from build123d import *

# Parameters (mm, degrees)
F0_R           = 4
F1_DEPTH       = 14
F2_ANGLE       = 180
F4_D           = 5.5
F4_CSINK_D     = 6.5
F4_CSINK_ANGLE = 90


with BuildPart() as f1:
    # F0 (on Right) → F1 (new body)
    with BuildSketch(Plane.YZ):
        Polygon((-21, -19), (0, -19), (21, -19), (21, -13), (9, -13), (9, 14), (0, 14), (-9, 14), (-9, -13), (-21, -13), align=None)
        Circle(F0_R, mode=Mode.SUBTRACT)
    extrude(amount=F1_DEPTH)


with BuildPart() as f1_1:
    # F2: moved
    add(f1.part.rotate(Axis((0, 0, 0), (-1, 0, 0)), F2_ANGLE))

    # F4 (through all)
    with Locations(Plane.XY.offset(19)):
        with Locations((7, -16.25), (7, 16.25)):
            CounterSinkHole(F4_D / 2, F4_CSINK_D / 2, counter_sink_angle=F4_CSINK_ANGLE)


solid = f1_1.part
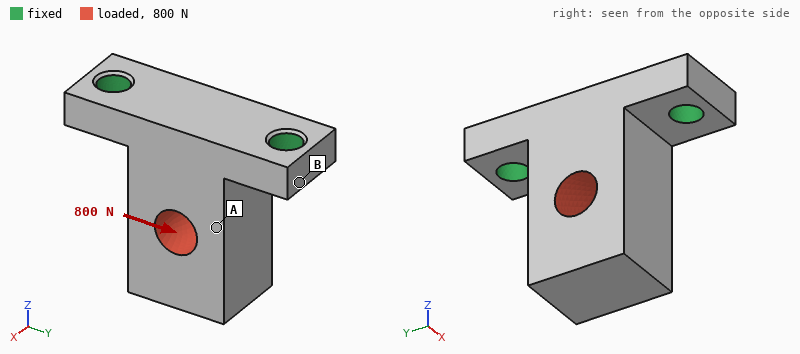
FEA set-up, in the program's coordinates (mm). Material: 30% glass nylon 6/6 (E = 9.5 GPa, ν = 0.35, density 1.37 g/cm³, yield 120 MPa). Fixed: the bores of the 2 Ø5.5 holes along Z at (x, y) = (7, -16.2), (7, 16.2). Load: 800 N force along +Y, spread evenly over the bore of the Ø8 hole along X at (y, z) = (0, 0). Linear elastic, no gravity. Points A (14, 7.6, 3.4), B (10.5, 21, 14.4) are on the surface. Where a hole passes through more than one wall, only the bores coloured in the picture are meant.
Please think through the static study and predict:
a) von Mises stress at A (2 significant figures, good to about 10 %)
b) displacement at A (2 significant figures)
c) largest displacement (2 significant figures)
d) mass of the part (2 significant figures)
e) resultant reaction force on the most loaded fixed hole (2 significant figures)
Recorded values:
6.8 MPa
0.054 mm
0.13 mm
13 g
660 N
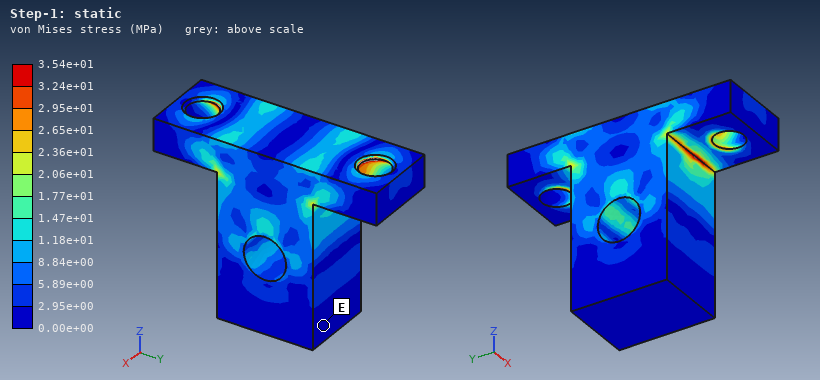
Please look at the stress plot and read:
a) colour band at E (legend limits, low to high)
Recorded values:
0.00e+00 to 2.95e+00 MPa
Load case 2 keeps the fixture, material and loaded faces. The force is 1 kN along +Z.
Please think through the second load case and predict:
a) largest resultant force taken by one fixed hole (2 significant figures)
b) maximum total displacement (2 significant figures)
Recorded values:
530 N
38 µm
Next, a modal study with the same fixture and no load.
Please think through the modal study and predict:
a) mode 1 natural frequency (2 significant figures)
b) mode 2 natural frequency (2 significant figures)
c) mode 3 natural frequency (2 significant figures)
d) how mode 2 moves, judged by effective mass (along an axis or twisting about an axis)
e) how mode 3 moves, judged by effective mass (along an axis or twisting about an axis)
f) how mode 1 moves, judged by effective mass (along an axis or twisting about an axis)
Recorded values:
2400 Hz
4900 Hz
8600 Hz
along Y
along Z
along X
